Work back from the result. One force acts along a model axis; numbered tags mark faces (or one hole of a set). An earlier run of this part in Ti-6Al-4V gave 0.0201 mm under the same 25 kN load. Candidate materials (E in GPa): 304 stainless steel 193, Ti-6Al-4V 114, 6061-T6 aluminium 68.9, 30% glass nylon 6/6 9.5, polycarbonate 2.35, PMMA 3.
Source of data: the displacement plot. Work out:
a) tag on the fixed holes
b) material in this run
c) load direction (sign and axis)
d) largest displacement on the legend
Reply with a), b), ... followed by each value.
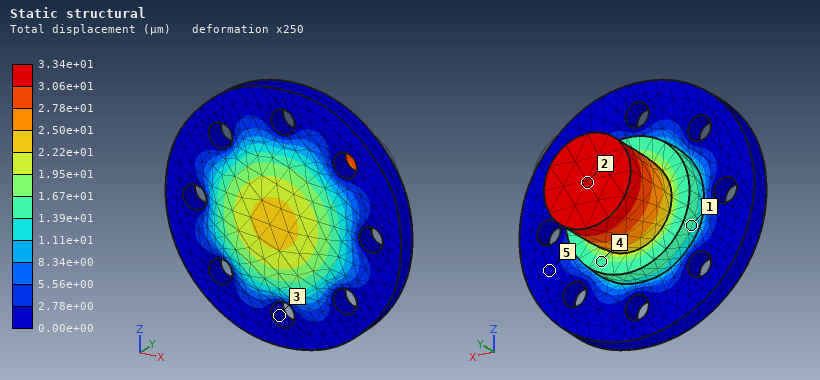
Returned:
a) 3
b) 6061-T6 aluminium
c) -Y
d) 3.34e+01 µm
